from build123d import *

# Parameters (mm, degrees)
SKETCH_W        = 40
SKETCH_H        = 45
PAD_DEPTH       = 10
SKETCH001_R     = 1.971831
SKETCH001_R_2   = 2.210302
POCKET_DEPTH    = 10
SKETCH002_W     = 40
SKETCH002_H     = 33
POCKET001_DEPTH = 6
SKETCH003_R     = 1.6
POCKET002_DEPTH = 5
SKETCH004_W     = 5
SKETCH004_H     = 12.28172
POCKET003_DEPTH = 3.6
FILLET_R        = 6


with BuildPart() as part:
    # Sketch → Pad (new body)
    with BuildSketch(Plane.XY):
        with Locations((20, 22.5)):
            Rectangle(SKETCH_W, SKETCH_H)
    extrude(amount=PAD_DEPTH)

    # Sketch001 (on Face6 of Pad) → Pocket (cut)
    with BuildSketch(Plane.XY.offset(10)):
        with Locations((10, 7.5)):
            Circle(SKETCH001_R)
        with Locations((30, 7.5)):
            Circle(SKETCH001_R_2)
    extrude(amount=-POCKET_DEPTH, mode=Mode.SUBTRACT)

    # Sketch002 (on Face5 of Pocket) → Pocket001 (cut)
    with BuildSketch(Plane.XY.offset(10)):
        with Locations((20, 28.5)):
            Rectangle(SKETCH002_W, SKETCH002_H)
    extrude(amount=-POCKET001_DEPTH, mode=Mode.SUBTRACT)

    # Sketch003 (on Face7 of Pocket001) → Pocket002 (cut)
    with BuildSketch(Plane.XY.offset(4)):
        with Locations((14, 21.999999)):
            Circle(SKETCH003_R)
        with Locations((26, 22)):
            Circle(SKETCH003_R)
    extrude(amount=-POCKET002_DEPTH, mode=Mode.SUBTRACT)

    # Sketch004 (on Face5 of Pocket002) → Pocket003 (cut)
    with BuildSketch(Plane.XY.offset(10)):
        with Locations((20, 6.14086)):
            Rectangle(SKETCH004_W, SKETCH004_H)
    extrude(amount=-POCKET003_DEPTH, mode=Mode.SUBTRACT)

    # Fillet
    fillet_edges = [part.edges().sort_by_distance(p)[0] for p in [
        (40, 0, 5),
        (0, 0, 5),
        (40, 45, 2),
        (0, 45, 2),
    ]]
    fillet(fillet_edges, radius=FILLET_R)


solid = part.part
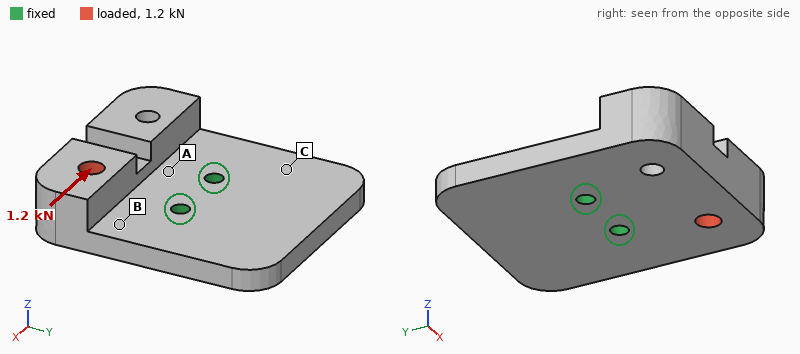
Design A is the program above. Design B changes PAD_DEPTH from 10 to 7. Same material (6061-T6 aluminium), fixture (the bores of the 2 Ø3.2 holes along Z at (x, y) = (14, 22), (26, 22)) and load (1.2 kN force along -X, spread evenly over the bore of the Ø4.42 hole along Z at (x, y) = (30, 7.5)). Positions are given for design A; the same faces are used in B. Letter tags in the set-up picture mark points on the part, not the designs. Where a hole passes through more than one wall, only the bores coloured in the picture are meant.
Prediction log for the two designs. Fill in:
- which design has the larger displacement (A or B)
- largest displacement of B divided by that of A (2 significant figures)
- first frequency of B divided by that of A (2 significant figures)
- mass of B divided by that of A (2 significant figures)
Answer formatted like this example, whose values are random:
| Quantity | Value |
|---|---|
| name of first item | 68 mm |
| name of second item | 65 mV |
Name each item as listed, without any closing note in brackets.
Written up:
| Quantity | Value |
|---|---|
| which design has the larger displacement | A |
| largest displacement of B divided by that of A | 0.69 |
| first frequency of B divided by that of A | 1.2 |
| mass of B divided by that of A | 0.88 |
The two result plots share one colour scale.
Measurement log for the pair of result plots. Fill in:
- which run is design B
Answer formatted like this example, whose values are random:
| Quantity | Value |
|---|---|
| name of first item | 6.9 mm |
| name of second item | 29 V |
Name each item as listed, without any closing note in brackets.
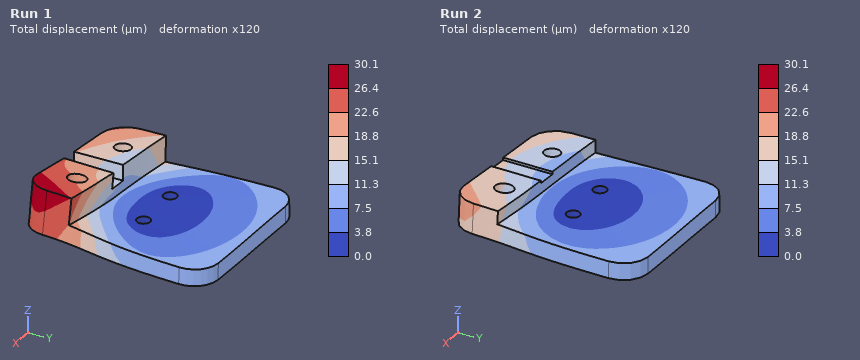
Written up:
| Quantity | Value |
|---|---|
| which run is design B | Run 2 |
